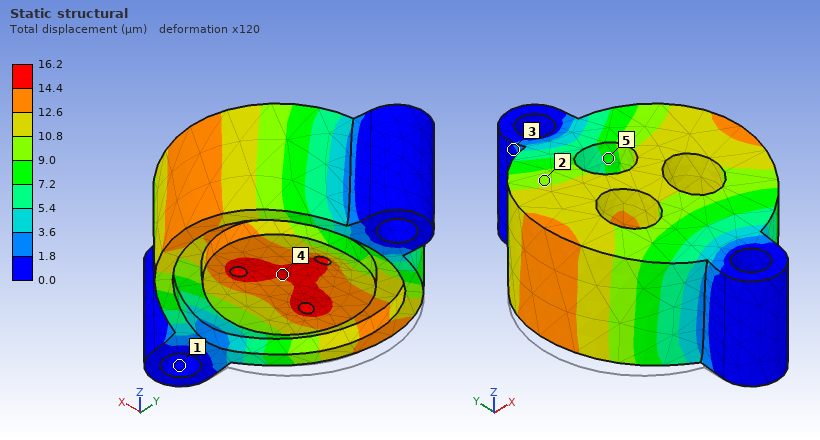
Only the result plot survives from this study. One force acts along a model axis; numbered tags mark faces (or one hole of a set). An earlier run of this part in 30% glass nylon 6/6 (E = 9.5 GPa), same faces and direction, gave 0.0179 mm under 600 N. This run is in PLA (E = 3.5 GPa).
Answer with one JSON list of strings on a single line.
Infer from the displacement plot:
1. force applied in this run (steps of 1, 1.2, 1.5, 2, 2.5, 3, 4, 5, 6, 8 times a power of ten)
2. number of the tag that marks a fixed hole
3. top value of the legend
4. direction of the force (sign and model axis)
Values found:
["200 N", "1", "16.2 µm", "+Z"]
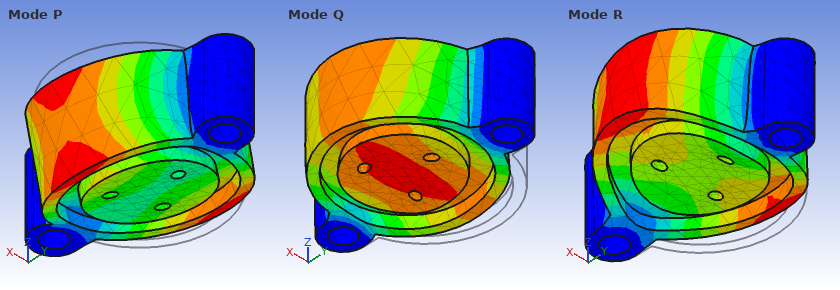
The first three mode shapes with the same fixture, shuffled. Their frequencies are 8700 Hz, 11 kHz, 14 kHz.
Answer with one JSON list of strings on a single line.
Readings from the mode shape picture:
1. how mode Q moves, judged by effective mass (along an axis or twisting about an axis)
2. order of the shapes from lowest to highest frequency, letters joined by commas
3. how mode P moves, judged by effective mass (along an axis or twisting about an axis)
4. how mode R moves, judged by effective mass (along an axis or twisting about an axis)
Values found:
["along X", "P, R, Q", "twisting about Y", "along Z"]
